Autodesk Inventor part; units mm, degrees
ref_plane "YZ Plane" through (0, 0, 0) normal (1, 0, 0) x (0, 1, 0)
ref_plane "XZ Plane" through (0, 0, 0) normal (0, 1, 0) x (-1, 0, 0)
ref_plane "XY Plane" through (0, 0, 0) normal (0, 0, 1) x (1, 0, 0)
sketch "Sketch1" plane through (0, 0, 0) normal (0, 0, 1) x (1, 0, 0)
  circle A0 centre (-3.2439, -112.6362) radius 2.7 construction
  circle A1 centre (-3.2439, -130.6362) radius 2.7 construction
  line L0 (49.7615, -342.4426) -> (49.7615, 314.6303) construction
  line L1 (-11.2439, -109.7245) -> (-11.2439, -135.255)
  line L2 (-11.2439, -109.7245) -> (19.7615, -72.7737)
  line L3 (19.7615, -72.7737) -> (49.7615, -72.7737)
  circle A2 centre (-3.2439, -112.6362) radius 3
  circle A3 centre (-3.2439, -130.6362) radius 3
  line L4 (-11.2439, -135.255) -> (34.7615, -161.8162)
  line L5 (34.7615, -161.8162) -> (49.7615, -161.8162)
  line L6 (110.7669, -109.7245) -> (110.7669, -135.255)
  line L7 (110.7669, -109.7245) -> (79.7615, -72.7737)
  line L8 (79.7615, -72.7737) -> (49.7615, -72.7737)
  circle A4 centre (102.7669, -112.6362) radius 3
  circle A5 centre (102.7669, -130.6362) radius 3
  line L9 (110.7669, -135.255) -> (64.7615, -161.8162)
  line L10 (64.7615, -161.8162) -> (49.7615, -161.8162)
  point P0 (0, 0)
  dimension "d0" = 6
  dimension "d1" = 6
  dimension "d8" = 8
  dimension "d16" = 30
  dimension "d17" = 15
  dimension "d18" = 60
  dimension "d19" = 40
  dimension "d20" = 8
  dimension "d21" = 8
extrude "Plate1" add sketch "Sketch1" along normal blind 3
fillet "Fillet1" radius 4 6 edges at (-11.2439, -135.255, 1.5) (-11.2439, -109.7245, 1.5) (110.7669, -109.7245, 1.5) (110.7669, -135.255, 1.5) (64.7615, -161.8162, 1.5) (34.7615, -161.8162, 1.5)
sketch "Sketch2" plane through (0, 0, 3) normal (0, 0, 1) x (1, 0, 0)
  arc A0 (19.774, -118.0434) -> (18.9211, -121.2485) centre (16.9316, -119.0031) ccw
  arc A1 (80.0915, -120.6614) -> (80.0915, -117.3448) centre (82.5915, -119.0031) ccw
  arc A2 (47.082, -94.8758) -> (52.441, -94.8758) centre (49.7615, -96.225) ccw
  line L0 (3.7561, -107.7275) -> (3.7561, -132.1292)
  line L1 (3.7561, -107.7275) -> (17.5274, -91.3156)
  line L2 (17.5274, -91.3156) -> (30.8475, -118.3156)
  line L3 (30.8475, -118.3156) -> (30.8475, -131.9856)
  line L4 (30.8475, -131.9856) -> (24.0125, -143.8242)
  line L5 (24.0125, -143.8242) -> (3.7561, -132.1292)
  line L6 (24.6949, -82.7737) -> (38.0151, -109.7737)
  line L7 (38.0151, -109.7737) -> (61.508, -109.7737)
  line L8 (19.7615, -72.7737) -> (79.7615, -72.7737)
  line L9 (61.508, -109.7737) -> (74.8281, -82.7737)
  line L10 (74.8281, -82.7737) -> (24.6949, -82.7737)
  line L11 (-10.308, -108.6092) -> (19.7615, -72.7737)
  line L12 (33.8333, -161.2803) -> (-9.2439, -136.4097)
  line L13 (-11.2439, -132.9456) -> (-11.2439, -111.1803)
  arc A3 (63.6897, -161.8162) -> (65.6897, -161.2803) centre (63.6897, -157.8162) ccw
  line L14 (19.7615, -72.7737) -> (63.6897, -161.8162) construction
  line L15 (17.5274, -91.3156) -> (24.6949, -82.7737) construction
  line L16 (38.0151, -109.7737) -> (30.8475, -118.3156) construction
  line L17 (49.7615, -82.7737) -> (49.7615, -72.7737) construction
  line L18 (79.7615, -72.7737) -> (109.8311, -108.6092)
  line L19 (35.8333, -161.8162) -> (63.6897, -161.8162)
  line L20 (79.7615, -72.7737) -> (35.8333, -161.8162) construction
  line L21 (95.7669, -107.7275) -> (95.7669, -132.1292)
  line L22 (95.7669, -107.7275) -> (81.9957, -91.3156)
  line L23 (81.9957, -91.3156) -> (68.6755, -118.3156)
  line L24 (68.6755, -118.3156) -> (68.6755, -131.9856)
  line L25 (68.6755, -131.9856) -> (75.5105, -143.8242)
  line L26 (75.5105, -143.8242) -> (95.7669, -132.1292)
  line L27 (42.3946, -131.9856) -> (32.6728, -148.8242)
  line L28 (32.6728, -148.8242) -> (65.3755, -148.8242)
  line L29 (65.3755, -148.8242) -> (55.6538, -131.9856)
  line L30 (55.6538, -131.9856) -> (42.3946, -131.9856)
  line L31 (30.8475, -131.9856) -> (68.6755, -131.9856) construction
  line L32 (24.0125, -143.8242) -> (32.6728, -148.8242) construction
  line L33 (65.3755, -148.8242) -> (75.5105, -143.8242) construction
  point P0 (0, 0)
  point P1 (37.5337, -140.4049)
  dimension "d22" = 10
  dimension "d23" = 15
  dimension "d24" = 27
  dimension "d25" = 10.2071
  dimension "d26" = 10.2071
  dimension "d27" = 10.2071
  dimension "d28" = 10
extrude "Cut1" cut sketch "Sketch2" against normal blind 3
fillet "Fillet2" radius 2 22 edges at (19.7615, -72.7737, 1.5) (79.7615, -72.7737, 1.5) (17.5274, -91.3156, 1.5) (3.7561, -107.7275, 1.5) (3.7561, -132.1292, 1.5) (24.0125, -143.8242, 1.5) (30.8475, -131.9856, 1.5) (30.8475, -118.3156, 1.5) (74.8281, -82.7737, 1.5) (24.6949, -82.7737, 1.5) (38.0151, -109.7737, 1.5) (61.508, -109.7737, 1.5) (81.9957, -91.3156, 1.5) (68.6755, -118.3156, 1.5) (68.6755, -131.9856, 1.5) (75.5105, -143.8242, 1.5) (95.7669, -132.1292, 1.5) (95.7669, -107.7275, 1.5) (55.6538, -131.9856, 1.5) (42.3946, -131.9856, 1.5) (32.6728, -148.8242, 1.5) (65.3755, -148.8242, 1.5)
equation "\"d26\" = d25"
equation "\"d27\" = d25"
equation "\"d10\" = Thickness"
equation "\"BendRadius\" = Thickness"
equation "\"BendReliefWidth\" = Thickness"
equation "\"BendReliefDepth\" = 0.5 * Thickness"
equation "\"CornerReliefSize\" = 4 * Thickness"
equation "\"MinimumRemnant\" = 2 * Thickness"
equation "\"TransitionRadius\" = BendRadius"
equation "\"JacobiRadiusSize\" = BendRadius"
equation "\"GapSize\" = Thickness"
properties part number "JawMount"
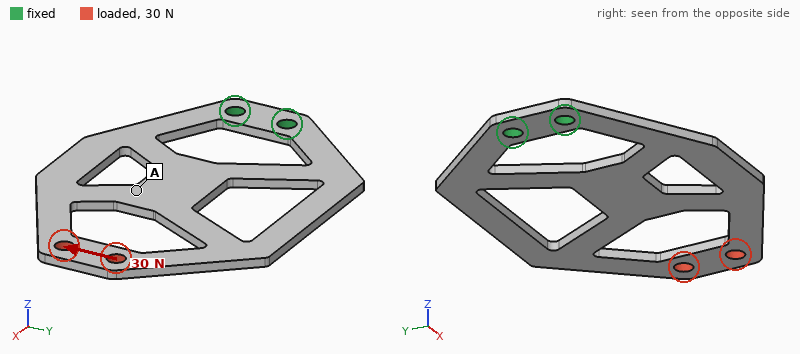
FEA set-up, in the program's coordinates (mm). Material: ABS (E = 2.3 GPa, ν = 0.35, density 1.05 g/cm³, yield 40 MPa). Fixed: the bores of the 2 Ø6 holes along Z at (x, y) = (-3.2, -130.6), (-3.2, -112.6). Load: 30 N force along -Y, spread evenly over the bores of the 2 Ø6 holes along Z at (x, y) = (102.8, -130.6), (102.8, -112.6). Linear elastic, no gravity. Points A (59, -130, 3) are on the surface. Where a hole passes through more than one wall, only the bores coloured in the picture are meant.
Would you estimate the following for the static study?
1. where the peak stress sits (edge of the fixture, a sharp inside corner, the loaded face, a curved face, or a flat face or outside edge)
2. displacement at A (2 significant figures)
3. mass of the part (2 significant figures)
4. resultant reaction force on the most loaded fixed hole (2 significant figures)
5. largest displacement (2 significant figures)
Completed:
a curved face
0.77 mm
16 g
92 N
1.4 mm
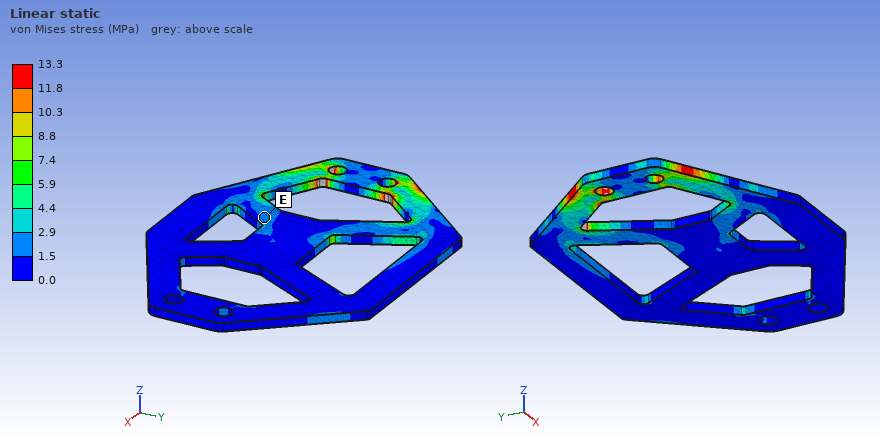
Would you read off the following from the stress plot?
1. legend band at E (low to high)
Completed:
1.5 to 2.9 MPa
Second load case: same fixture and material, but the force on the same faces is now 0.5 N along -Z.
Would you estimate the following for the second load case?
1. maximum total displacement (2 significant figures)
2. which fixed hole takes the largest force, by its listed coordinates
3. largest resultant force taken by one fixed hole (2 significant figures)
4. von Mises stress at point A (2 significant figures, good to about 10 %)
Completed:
1.8 mm
(-3.2, -130.6)
0.39 N
0.27 MPa
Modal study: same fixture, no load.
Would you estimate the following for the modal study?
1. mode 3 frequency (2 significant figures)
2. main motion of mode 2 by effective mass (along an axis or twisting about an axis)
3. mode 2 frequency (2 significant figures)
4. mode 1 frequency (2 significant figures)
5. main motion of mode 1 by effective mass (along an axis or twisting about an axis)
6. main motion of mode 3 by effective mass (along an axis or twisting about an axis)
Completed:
260 Hz
twisting about X
130 Hz
42 Hz
along Z
along Z
